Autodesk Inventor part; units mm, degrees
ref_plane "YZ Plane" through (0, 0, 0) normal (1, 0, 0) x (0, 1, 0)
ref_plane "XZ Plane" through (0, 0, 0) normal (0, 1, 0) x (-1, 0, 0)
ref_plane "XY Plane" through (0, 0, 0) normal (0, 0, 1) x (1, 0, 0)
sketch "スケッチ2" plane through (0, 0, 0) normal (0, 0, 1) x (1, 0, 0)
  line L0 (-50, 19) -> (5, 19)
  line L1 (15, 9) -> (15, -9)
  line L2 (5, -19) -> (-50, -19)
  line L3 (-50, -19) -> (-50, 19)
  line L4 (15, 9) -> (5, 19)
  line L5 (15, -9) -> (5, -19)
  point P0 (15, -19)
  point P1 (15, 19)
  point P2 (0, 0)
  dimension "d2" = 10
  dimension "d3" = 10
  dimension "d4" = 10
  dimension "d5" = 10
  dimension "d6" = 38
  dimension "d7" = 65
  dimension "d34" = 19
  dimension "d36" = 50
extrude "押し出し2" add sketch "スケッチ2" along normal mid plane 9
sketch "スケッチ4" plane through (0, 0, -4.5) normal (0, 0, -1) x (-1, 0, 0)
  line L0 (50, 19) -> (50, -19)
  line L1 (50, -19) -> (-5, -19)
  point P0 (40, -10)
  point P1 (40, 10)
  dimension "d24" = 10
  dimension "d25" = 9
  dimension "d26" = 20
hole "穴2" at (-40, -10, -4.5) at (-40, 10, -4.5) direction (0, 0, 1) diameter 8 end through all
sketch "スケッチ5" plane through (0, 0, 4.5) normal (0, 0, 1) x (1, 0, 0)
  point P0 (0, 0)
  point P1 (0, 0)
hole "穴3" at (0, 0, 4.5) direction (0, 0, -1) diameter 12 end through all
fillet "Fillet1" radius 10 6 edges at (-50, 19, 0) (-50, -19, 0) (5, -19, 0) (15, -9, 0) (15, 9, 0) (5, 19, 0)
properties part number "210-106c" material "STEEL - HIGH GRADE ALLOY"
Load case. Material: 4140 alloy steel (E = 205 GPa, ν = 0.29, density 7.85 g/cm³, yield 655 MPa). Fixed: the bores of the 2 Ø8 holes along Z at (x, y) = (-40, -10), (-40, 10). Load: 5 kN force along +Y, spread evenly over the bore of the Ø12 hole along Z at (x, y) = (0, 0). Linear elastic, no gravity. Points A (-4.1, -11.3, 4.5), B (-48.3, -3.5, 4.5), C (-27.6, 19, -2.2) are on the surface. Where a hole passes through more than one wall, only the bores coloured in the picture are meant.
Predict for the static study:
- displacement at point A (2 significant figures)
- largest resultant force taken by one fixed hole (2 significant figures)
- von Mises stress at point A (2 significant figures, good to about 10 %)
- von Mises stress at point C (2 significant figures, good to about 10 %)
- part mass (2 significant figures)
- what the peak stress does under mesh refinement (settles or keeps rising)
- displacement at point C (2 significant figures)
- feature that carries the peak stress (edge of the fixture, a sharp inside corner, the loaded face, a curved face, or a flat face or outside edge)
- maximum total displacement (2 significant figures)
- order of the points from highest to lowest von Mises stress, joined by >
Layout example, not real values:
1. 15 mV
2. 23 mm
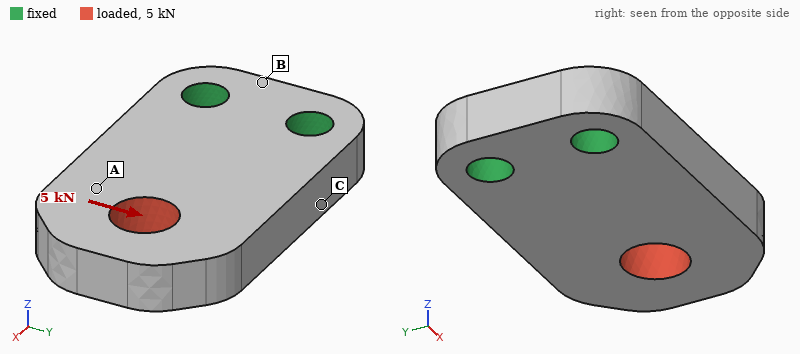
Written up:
1. 19 µm
2. 8.0 kN
3. 30 MPa
4. 57 MPa
5. 150 g
6. keeps rising
7. 7.2 µm
8. edge of the fixture
9. 31 µm
10. C > A > B
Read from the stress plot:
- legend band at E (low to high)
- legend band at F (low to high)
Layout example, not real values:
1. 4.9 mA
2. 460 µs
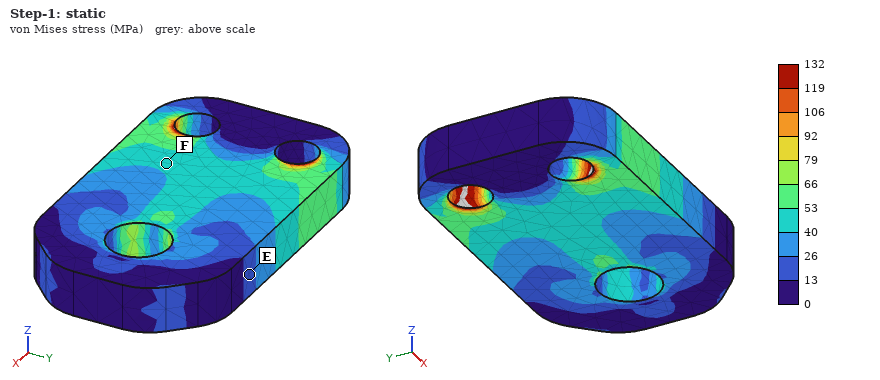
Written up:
1. 13 to 26 MPa
2. 40 to 53 MPa
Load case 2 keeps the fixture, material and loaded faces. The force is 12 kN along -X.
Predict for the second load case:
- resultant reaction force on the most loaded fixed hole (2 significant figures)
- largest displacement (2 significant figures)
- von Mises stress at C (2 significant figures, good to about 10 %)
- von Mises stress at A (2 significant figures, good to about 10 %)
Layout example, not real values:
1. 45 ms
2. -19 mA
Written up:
1. 6.0 kN
2. 11 µm
3. 30 MPa
4. 40 MPa
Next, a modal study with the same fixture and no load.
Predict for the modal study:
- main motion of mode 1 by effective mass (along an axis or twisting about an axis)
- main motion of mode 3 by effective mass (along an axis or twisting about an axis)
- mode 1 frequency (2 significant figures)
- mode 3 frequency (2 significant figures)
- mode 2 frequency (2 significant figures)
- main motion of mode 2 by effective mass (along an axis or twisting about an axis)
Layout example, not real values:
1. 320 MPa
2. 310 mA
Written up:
1. along Z
2. along Y
3. 3000 Hz
4. 8900 Hz
5. 8300 Hz
6. twisting about X
